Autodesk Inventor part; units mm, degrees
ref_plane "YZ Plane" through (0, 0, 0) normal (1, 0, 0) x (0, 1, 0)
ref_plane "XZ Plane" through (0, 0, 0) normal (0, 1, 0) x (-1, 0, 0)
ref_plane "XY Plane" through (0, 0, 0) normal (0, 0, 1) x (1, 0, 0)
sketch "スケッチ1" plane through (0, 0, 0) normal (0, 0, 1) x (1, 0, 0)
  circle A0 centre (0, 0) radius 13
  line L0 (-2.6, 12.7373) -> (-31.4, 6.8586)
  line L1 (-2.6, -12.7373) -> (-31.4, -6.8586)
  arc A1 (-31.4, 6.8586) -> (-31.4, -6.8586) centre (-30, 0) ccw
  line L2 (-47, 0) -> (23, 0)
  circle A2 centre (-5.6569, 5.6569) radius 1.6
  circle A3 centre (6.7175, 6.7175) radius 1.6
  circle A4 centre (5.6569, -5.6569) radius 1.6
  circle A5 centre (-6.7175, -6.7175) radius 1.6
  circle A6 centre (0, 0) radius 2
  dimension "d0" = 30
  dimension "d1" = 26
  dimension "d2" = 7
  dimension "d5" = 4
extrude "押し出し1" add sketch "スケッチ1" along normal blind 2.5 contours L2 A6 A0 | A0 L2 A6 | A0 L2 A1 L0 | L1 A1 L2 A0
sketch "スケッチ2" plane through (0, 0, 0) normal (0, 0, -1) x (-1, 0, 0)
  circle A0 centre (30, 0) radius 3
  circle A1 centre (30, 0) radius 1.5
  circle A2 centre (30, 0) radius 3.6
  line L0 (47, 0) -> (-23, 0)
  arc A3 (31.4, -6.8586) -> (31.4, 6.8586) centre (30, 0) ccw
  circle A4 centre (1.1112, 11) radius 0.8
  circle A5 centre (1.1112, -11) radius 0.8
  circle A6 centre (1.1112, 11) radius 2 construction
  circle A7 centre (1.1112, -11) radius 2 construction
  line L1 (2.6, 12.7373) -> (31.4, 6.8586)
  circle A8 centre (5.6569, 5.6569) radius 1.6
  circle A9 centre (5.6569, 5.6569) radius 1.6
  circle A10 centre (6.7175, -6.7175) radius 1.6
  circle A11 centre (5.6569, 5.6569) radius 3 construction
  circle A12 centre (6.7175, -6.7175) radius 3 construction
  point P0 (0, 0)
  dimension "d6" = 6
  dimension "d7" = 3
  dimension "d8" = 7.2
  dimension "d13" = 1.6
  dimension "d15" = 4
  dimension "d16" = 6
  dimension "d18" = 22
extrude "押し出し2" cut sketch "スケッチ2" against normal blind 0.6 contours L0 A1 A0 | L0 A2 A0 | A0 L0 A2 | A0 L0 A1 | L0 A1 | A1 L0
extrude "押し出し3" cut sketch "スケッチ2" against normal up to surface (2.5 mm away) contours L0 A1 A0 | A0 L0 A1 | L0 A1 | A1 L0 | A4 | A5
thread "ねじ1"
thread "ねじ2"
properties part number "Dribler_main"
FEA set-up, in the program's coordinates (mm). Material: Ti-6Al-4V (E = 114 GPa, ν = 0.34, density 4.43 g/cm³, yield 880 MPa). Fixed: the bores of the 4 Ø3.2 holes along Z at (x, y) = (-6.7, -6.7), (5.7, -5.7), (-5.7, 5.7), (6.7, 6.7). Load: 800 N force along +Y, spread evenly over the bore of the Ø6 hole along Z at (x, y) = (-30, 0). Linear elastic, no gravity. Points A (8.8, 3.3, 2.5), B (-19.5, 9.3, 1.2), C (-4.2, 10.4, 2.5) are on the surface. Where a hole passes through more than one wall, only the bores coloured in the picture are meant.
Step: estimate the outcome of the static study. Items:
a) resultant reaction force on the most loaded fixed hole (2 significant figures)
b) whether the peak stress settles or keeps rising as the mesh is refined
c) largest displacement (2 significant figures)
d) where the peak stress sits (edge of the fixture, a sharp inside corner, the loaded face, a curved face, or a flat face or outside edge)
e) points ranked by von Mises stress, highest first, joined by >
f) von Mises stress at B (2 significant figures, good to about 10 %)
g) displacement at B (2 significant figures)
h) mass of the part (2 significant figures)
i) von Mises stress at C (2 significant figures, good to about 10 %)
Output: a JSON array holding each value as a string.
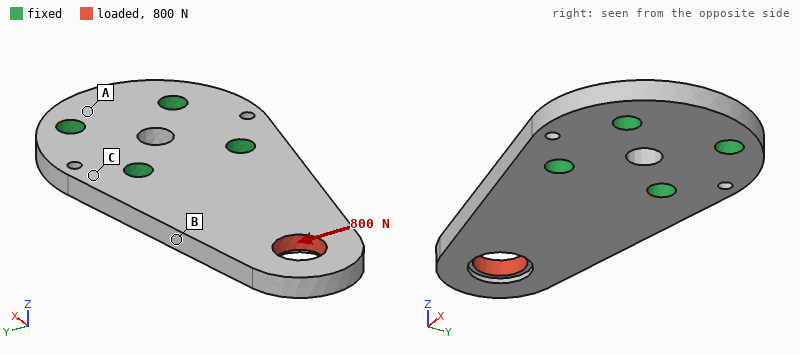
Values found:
["1.2 kN", "keeps rising", "41 µm", "edge of the fixture", "B > C > A", "66 MPa", "15 µm", "9.7 g", "29 MPa"]
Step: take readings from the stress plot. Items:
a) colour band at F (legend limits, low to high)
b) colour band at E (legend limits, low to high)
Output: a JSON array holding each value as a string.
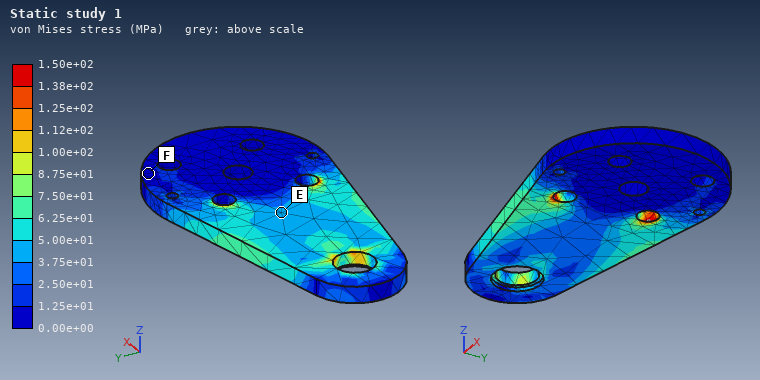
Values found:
["0.00e+00 to 1.25e+01 MPa", "3.75e+01 to 5.00e+01 MPa"]
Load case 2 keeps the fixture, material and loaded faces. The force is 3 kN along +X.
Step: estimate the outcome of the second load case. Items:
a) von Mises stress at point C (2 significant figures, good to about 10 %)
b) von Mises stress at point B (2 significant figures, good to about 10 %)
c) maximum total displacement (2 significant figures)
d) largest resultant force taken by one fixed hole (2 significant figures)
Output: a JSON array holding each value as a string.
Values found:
["27 MPa", "66 MPa", "0.14 mm", "1.4 kN"]
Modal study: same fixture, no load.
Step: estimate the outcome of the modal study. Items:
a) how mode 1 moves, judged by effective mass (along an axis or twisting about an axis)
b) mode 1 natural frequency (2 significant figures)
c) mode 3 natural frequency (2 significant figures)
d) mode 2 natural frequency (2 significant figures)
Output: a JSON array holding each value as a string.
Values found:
["along Z", "3200 Hz", "15 kHz", "11 kHz"]
